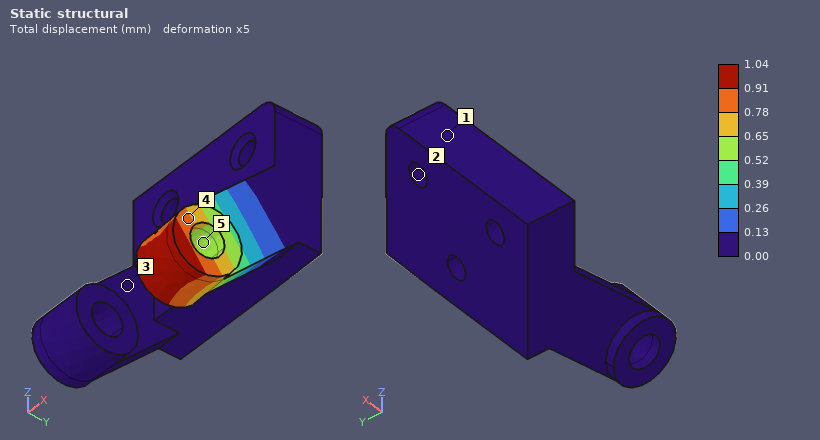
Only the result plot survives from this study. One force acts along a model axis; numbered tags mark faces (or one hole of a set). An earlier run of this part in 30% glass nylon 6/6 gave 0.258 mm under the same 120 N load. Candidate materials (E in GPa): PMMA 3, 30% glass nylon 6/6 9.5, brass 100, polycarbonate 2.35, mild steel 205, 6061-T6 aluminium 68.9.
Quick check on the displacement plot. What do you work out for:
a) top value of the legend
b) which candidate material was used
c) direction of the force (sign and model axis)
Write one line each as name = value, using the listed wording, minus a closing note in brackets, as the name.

top value of the legend = 1.04 mm
which candidate material was used = polycarbonate
direction of the force = -X
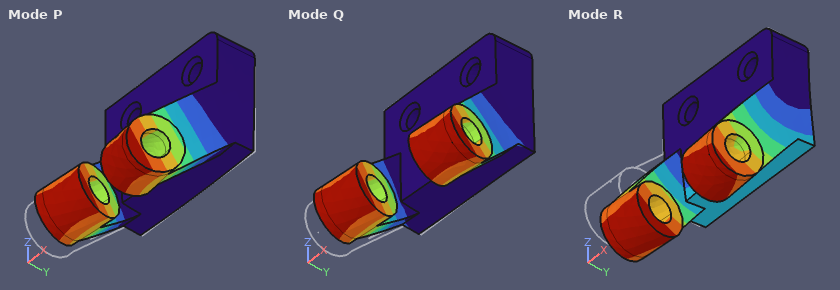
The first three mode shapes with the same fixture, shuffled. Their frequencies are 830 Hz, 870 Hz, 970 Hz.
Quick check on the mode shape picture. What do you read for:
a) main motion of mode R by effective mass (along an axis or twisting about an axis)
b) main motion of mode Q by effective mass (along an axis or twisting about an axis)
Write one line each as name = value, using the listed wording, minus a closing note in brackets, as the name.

main motion of mode R by effective mass = along Y
main motion of mode Q by effective mass = along X
